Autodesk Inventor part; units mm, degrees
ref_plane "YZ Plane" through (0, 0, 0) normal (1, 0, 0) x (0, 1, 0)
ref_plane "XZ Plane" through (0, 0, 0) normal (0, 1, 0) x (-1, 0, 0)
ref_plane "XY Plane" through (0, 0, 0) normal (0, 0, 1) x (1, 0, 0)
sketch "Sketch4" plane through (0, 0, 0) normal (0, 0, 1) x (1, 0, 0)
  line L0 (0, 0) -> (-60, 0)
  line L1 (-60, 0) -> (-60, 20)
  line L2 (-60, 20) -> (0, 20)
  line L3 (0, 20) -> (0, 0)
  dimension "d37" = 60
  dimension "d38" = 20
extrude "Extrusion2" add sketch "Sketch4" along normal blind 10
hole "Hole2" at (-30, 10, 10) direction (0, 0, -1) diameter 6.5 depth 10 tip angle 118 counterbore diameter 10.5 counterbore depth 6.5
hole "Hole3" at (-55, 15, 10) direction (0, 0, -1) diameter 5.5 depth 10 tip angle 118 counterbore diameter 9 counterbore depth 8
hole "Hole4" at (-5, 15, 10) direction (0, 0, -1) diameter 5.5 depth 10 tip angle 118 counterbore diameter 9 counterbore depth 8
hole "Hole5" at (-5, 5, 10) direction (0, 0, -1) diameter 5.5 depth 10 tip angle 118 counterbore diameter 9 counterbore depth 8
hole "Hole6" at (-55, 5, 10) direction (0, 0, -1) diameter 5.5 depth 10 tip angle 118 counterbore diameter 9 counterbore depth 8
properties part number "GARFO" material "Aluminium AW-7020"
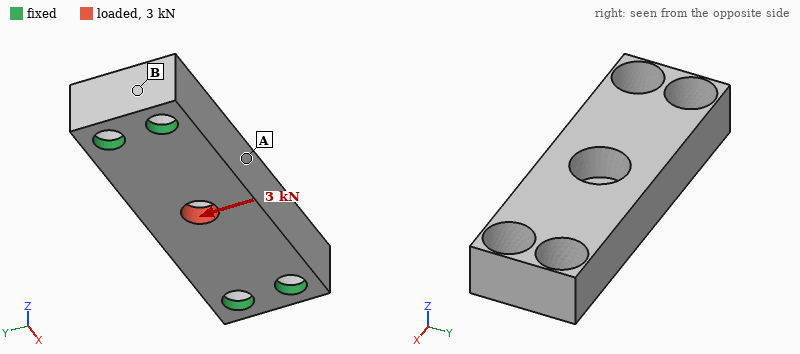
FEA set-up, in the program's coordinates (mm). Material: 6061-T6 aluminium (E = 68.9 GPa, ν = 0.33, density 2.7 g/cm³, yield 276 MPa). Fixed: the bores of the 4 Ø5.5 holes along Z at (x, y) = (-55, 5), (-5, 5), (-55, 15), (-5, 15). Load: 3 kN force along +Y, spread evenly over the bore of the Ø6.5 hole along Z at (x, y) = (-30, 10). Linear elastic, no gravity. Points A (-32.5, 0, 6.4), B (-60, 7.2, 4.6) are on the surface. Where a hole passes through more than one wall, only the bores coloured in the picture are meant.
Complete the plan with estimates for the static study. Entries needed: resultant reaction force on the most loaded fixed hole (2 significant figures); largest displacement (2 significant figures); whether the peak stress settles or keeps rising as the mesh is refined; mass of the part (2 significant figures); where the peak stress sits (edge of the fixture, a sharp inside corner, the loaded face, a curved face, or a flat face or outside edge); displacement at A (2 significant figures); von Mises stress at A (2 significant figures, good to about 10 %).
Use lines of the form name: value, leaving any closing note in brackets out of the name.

resultant reaction force on the most loaded fixed hole: 1.0 kN
largest displacement: 25 µm
whether the peak stress settles or keeps rising as the mesh is refined: keeps rising
mass of the part: 25 g
where the peak stress sits: edge of the fixture
displacement at A: 17 µm
von Mises stress at A: 39 MPa
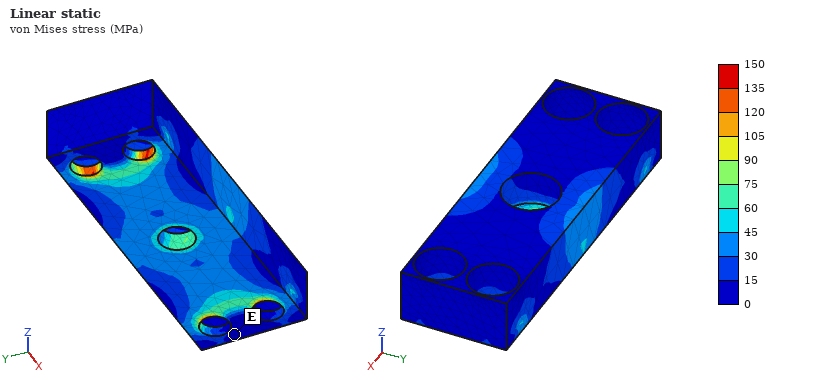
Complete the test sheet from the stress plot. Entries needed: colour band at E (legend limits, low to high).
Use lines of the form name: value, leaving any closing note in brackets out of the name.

colour band at E: 0 to 15 MPa
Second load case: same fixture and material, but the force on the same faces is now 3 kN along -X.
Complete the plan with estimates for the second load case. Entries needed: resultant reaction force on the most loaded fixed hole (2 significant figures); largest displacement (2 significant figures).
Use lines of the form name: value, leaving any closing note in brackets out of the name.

resultant reaction force on the most loaded fixed hole: 760 N
largest displacement: 8.9 µm
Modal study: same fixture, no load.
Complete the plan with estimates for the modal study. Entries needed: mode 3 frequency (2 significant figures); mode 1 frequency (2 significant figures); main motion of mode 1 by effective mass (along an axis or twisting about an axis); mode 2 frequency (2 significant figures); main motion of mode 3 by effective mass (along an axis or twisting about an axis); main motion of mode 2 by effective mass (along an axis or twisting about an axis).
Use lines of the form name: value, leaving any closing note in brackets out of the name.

mode 3 frequency: 21 kHz
mode 1 frequency: 12 kHz
main motion of mode 1 by effective mass: along Z
mode 2 frequency: 15 kHz
main motion of mode 3 by effective mass: along Y
main motion of mode 2 by effective mass: along Y
